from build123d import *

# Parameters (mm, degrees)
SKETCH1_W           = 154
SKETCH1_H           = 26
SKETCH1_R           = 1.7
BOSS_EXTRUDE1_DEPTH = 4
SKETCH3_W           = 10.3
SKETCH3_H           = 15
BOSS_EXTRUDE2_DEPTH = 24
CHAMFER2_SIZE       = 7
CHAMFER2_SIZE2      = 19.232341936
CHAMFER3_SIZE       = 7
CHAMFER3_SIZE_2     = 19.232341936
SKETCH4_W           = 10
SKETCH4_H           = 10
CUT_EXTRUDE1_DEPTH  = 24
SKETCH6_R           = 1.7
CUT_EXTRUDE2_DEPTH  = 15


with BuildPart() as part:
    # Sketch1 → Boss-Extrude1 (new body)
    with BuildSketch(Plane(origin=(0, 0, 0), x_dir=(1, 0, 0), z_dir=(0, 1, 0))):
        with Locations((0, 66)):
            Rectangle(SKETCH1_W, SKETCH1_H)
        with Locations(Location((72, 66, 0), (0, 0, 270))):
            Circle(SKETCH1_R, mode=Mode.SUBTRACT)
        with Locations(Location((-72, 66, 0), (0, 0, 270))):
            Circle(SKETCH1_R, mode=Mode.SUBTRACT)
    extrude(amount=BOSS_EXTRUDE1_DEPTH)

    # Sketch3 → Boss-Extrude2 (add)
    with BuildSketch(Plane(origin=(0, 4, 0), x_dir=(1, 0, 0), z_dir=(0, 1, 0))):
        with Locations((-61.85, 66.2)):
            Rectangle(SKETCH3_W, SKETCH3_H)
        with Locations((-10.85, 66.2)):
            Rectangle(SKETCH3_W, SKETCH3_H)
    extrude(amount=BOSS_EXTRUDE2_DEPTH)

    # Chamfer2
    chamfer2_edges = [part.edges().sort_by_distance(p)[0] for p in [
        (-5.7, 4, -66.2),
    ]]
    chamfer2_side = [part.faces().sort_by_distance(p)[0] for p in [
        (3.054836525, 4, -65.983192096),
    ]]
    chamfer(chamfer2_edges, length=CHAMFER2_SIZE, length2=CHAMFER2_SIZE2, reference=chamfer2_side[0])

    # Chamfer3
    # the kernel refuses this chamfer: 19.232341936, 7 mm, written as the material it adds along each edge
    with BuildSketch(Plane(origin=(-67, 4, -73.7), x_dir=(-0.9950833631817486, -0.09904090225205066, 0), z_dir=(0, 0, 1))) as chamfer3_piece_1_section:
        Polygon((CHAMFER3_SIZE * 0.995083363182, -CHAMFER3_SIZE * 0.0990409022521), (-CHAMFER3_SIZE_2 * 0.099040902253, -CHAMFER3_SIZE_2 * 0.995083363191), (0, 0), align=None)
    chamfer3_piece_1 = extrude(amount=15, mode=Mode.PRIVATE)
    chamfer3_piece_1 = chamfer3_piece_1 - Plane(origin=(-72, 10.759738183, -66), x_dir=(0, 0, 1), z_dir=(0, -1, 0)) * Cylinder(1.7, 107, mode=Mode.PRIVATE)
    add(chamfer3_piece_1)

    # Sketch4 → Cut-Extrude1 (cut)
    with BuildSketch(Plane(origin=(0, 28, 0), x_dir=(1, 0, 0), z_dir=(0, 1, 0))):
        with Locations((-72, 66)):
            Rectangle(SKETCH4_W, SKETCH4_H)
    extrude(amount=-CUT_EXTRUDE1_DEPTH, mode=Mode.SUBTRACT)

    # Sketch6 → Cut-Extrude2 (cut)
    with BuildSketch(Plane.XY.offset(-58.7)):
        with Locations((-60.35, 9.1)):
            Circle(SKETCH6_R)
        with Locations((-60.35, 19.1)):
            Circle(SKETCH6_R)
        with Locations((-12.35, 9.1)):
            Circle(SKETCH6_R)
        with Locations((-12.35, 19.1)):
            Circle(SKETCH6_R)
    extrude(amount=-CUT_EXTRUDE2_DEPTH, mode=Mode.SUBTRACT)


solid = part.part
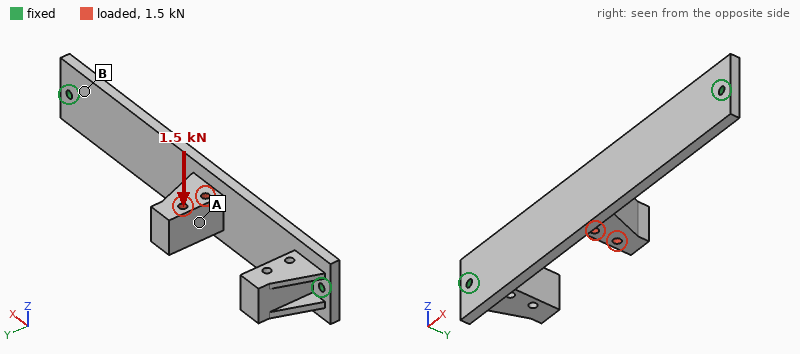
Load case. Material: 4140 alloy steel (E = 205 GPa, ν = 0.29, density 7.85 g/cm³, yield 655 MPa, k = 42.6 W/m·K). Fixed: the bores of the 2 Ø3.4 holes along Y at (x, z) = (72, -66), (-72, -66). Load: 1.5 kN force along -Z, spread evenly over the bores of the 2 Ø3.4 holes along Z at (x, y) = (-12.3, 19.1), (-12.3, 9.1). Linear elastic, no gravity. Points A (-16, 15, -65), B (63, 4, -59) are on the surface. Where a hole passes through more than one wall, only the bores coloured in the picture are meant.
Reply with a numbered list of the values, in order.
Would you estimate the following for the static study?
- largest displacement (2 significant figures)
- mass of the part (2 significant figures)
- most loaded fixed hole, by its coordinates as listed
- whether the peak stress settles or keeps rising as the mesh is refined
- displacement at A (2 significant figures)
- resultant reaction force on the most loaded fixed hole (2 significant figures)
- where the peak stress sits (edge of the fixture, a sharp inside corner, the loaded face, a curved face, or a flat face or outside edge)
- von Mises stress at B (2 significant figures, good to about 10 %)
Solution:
1. 0.39 mm
2. 190 g
3. (-72, -66)
4. keeps rising
5. 0.22 mm
6. 890 N
7. edge of the fixture
8. 89 MPa
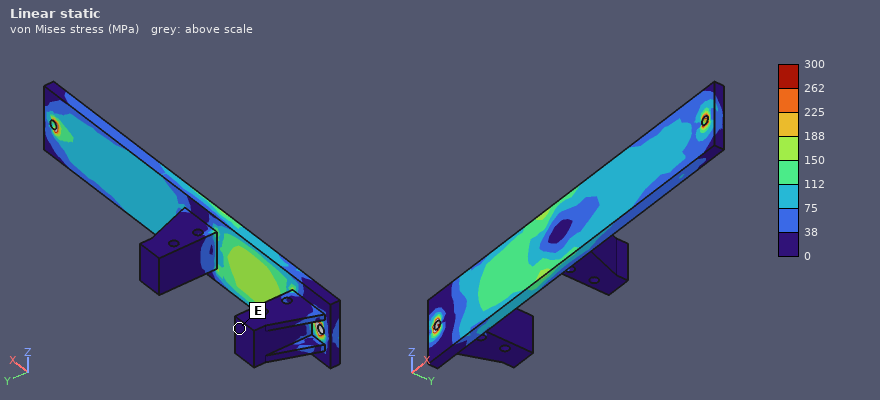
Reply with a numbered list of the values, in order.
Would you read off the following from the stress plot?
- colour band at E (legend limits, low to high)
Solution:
1. 0 to 38 MPa
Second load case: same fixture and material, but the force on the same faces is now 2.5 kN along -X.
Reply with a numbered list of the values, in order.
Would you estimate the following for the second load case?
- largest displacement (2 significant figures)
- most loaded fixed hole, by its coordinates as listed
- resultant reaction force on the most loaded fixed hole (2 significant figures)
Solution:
1. 0.21 mm
2. (-72, -66)
3. 1.4 kN
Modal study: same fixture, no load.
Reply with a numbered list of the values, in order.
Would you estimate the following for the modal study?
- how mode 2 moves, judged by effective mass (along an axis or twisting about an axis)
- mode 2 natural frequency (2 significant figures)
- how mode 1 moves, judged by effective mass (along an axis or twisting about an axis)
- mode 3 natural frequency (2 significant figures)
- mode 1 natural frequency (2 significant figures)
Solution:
1. along Z
2. 1700 Hz
3. along Y
4. 2200 Hz
5. 860 Hz
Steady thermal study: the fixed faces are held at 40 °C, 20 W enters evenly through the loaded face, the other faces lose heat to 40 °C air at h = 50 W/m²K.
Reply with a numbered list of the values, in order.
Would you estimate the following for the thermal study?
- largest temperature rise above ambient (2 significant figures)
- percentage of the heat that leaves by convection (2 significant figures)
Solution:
1. 79 K
2. 79 %
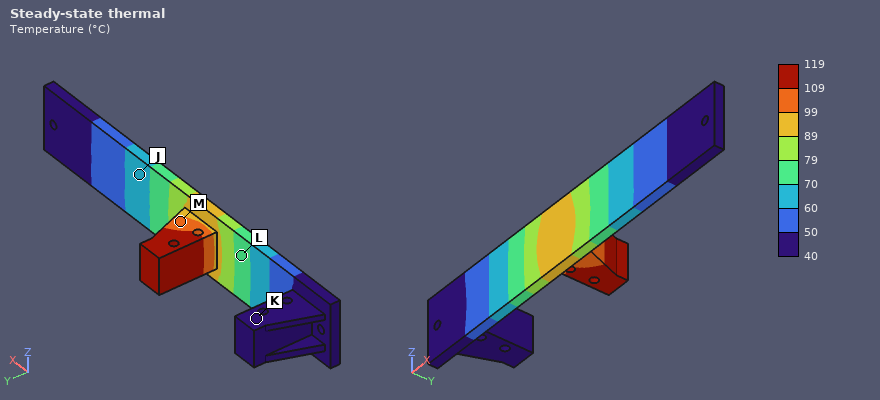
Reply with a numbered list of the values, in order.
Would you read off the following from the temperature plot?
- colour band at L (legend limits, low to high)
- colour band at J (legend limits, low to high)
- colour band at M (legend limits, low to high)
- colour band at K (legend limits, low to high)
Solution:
1. 70 to 79 °C
2. 60 to 70 °C
3. 99 to 109 °C
4. 40 to 50 °C
